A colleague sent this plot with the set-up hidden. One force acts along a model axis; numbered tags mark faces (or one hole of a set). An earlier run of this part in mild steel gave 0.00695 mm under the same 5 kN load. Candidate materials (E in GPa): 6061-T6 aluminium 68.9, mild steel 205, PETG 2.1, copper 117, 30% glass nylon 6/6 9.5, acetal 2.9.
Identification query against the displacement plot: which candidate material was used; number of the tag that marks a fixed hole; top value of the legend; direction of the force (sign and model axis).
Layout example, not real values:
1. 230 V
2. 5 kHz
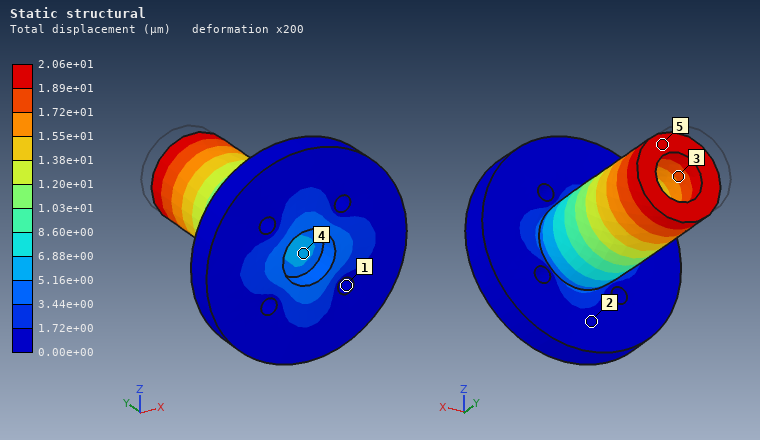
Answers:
1. 6061-T6 aluminium
2. 1
3. 2.06e+01 µm
4. -Y
